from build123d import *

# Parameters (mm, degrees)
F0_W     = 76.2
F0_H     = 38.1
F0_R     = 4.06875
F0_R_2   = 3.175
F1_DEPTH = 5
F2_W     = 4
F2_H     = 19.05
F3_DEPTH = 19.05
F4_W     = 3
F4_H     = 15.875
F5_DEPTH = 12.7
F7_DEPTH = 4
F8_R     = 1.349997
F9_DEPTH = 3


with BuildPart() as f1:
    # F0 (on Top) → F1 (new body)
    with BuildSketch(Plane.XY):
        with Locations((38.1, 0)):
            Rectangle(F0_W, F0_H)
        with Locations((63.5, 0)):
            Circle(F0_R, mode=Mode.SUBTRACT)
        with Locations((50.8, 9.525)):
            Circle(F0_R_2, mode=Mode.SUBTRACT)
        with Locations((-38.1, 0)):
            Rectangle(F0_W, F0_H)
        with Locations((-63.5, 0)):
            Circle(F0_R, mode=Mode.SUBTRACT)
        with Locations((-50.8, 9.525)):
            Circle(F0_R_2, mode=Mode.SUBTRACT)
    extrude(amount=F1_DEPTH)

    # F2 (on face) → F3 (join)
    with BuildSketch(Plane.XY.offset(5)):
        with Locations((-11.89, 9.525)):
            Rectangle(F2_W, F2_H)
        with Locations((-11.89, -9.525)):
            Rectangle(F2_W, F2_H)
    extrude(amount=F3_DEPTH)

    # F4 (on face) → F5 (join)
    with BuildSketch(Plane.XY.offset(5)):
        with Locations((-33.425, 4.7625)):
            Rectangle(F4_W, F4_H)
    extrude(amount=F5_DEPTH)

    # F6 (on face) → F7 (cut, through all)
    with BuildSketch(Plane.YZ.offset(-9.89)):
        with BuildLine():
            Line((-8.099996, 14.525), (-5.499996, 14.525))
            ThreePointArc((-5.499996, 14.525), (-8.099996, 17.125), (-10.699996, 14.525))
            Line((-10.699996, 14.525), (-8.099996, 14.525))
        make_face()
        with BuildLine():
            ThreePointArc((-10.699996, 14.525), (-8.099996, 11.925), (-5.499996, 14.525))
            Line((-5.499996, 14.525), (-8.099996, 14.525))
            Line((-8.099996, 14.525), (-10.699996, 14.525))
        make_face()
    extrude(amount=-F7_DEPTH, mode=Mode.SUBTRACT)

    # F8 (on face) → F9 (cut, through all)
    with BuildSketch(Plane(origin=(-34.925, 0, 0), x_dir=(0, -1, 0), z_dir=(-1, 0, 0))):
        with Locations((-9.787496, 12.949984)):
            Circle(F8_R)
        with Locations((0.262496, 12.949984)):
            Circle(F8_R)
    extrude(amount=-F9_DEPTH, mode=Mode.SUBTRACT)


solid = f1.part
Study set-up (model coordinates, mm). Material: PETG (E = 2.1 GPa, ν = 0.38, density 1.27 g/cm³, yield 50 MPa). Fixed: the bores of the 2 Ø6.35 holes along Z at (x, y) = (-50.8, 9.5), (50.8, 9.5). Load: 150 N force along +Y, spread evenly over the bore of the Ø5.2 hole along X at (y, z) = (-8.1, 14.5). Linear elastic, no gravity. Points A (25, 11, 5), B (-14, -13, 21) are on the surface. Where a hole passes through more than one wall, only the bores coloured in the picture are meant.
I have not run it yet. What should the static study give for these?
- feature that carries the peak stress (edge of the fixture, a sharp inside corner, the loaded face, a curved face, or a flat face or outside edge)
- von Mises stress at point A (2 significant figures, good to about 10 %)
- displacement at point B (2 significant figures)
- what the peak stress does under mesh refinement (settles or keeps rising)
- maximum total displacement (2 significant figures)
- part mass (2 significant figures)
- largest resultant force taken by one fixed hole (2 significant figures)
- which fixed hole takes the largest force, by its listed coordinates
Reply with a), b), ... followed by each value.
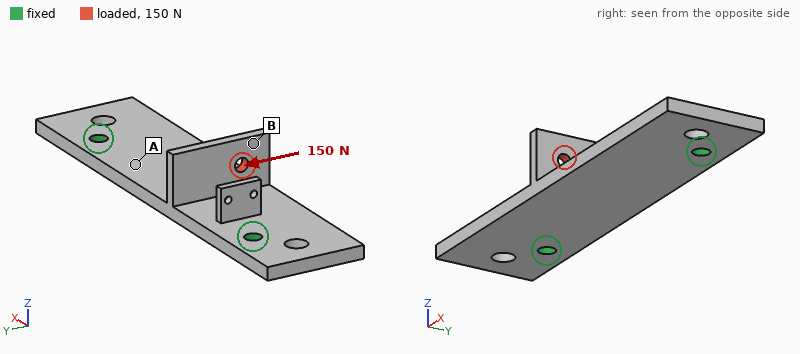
a) edge of the fixture
b) 4.6 MPa
c) 0.90 mm
d) keeps rising
e) 1.1 mm
f) 40 g
g) 110 N
h) (-50.8, 9.5)
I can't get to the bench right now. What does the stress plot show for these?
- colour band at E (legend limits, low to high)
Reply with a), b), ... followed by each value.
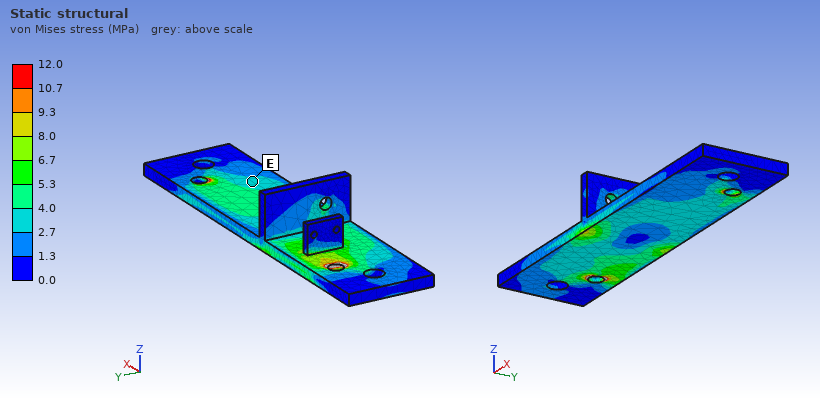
a) 2.7 to 4.0 MPa
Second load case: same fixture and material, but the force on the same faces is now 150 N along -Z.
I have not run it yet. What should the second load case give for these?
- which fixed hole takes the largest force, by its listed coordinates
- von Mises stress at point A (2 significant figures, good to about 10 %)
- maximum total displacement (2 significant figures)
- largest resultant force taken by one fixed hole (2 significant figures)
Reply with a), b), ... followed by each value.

a) (-50.8, 9.5)
b) 3.1 MPa
c) 1.9 mm
d) 99 N
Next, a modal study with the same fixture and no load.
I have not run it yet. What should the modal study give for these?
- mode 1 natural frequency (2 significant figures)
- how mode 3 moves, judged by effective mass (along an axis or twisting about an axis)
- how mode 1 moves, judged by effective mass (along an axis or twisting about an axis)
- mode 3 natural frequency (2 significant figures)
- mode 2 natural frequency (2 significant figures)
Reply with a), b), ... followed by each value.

a) 490 Hz
b) twisting about Y
c) along Z
d) 1100 Hz
e) 750 Hz
